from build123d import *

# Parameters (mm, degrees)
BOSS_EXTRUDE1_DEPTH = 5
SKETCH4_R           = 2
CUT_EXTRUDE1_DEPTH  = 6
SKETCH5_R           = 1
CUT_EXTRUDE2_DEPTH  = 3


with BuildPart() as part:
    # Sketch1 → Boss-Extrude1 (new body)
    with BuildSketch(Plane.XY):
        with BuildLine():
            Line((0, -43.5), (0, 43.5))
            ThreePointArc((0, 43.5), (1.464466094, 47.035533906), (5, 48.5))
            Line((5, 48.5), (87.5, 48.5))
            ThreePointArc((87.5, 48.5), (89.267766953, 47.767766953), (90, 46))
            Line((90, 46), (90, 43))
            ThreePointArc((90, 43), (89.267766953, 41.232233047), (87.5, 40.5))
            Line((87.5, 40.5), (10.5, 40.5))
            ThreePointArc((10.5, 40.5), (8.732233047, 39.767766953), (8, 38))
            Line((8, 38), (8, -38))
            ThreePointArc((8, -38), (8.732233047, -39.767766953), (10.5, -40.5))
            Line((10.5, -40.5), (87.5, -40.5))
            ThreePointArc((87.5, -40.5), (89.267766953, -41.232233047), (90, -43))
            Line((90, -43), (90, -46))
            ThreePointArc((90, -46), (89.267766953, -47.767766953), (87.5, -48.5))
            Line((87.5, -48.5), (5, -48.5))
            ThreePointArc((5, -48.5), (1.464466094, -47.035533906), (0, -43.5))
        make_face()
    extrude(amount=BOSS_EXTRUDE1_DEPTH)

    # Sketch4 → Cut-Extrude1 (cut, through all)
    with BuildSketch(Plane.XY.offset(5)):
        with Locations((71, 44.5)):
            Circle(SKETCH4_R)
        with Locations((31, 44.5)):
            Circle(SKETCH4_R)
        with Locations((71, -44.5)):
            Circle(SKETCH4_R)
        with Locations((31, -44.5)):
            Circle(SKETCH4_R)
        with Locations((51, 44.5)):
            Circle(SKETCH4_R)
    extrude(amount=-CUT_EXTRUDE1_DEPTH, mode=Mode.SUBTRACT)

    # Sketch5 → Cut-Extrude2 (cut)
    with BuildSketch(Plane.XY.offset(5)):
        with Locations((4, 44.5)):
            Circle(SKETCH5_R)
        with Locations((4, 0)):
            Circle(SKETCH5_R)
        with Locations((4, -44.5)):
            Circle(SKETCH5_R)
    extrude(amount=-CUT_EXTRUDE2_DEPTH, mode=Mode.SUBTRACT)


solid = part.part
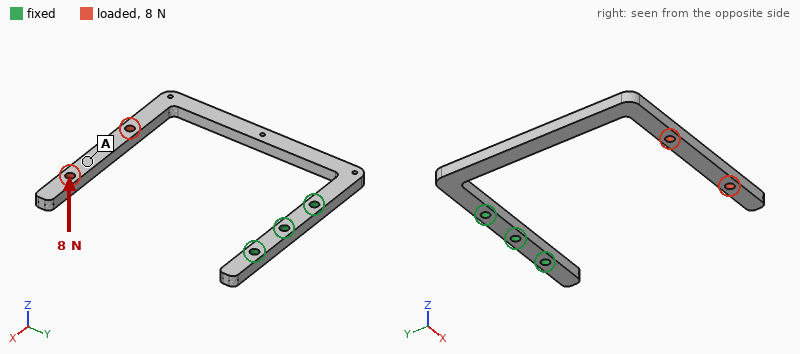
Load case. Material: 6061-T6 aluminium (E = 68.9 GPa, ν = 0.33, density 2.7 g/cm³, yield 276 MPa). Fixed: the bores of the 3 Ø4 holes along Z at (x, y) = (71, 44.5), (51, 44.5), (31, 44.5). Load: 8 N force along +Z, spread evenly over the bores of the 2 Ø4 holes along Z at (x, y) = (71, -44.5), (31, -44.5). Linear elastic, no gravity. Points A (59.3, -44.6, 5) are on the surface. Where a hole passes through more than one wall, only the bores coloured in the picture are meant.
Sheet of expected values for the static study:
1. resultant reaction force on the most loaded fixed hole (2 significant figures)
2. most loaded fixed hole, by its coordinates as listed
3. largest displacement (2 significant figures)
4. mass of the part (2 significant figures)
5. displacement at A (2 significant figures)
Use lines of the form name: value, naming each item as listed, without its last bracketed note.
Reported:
resultant reaction force on the most loaded fixed hole: 7.8 N
most loaded fixed hole, by its coordinates as listed: (31, 44.5)
largest displacement: 1.3 mm
mass of the part: 27 g
displacement at A: 1.0 mm
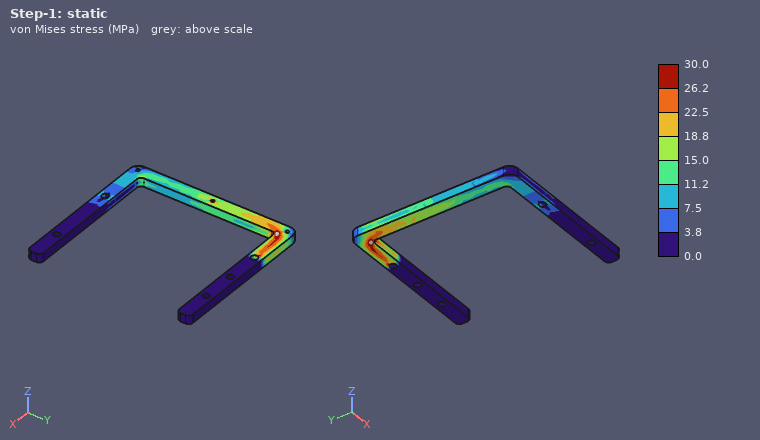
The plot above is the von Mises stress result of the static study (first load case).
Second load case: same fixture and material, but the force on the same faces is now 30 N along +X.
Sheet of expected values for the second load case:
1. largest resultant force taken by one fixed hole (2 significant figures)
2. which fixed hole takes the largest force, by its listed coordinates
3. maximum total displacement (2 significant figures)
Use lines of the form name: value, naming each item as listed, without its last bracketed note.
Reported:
largest resultant force taken by one fixed hole: 38 N
which fixed hole takes the largest force, by its listed coordinates: (31, 44.5)
maximum total displacement: 1.3 mm
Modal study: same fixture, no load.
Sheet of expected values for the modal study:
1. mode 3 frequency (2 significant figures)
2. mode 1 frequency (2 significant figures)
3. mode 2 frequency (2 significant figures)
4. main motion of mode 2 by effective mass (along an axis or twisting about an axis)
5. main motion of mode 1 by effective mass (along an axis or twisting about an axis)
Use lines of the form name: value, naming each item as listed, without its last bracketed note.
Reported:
mode 3 frequency: 380 Hz
mode 1 frequency: 150 Hz
mode 2 frequency: 240 Hz
main motion of mode 2 by effective mass: along X
main motion of mode 1 by effective mass: along Z
